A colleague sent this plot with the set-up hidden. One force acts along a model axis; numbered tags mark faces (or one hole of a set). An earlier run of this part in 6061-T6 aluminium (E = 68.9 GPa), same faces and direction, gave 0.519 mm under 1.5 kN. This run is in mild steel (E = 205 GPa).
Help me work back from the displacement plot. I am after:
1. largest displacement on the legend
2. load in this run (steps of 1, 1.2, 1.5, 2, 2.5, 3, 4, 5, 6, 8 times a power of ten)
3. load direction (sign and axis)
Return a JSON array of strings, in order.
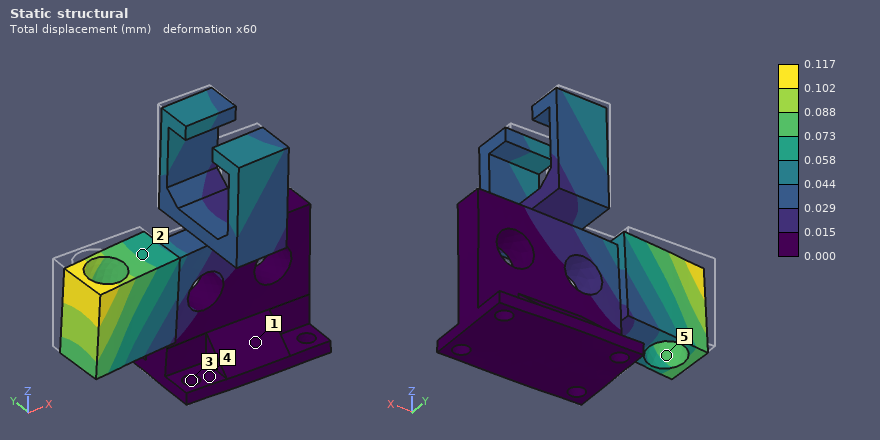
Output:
["0.117 mm", "1 kN", "-Y"]
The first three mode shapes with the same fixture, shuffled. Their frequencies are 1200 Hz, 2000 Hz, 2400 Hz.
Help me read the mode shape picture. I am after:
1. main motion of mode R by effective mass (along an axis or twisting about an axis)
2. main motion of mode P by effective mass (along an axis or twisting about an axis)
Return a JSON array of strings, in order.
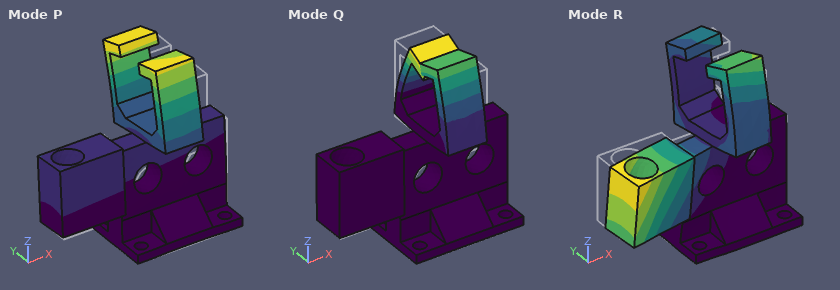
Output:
["along Y", "along Y"]
